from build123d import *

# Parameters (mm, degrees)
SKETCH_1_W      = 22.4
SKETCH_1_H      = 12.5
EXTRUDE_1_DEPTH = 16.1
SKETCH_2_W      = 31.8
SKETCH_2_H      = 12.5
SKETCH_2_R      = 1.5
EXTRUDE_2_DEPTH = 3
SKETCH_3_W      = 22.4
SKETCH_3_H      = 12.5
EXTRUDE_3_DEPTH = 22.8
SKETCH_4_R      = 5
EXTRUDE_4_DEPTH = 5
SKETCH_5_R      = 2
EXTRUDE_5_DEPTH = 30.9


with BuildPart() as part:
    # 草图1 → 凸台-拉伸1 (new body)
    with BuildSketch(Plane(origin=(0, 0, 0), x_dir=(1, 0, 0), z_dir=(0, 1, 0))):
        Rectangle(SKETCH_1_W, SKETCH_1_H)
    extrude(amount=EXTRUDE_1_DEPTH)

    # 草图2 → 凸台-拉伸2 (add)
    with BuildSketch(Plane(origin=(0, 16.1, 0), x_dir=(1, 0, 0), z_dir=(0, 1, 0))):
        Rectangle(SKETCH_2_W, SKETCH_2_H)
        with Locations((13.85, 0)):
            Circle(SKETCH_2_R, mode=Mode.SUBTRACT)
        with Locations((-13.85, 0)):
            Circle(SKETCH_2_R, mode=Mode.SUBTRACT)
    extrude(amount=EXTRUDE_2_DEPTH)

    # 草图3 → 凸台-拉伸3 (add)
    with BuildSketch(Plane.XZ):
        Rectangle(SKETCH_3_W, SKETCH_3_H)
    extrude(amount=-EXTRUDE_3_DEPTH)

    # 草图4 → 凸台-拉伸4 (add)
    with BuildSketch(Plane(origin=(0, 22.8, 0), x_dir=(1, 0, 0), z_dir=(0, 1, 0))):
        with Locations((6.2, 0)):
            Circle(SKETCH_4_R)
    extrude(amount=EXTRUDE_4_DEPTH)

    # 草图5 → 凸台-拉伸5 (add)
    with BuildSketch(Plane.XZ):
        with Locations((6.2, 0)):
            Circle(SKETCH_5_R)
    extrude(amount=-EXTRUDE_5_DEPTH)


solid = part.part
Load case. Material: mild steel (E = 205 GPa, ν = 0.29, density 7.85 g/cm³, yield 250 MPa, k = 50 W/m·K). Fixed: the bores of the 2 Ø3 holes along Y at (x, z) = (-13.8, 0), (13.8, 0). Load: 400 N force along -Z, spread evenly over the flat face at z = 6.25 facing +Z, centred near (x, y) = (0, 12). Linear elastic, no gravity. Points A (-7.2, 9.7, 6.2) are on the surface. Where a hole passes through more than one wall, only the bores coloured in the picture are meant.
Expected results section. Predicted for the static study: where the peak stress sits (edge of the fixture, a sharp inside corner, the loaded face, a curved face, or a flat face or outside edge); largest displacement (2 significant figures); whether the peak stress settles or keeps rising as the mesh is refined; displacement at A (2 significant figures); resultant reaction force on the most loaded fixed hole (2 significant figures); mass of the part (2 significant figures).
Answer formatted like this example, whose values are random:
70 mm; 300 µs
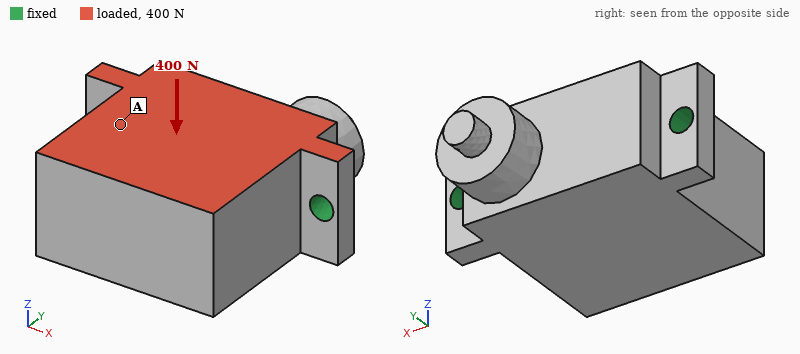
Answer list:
edge of the fixture; 8.0 µm; keeps rising; 4.4 µm; 200 N; 56 g
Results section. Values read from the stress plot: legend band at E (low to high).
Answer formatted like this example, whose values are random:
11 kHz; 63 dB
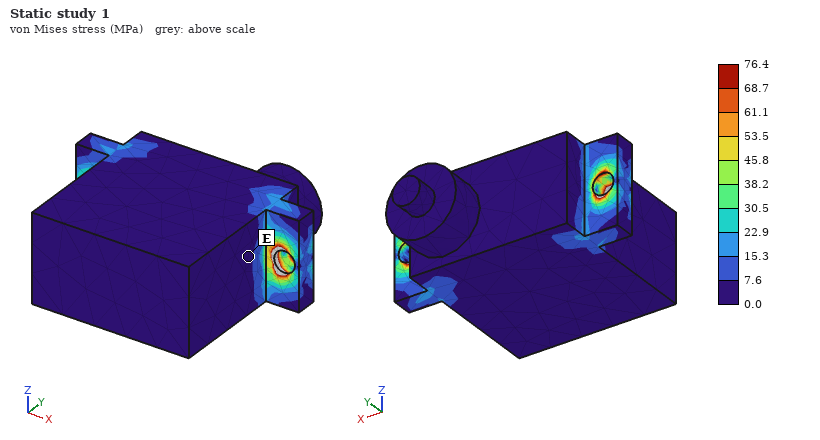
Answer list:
0.0 to 7.6 MPa
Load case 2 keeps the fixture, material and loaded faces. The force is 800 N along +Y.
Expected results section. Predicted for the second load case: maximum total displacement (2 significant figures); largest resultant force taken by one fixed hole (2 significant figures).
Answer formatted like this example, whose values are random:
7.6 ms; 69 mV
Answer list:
16 µm; 400 N
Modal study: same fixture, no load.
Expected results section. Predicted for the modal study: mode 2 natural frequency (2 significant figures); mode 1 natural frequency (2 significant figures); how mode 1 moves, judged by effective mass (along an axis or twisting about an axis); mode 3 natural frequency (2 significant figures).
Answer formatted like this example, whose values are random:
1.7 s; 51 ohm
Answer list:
19 kHz; 5400 Hz; along Z; 19 kHz
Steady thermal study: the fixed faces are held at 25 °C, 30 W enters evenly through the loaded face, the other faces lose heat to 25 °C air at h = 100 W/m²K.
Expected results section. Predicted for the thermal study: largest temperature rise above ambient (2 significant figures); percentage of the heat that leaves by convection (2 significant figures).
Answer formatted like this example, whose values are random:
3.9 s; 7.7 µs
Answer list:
44 K; 20 %
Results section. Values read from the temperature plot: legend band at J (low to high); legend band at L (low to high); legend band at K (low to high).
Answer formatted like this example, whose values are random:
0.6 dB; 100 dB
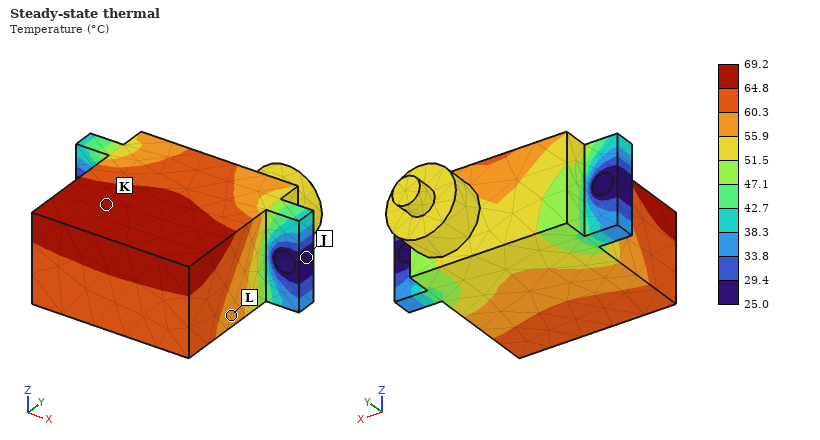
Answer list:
25.0 to 29.4 °C; 55.9 to 60.3 °C; 64.8 to 69.2 °C
